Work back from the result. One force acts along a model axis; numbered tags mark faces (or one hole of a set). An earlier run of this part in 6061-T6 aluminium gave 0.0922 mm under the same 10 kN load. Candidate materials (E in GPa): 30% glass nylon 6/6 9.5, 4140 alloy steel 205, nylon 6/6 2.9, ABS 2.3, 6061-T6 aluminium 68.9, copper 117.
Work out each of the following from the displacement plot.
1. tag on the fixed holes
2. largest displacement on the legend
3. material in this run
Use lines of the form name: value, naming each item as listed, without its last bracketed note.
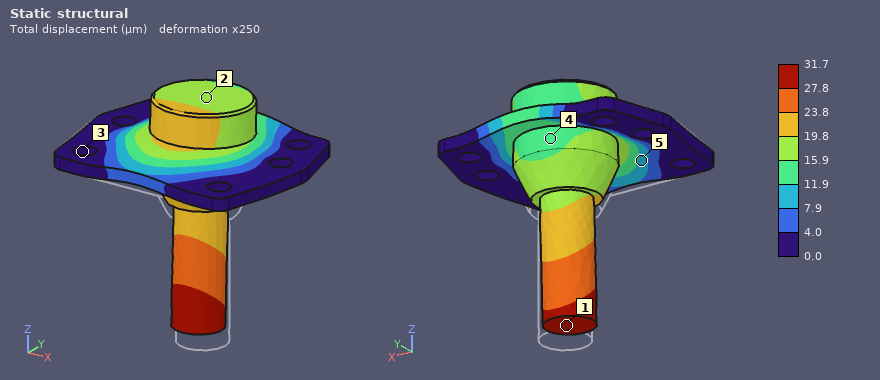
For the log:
tag on the fixed holes: 3
largest displacement on the legend: 31.7 µm
material in this run: 4140 alloy steel
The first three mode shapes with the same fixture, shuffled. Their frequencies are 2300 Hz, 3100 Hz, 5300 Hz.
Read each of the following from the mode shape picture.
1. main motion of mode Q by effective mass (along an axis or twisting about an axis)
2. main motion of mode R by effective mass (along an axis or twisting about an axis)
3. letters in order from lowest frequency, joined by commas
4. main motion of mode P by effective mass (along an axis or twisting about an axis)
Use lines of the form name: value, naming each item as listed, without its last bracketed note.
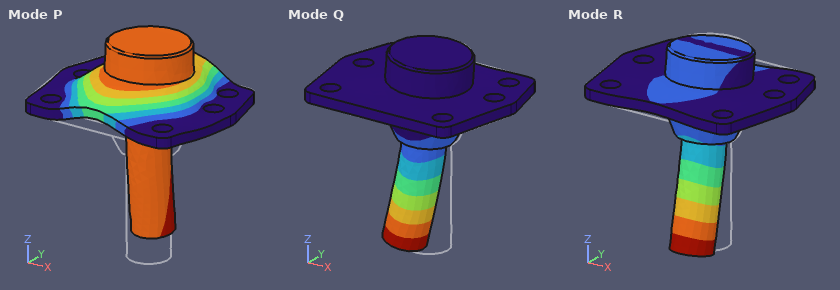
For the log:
main motion of mode Q by effective mass: along X
main motion of mode R by effective mass: along Y
letters in order from lowest frequency, joined by commas: R, Q, P
main motion of mode P by effective mass: along Z
